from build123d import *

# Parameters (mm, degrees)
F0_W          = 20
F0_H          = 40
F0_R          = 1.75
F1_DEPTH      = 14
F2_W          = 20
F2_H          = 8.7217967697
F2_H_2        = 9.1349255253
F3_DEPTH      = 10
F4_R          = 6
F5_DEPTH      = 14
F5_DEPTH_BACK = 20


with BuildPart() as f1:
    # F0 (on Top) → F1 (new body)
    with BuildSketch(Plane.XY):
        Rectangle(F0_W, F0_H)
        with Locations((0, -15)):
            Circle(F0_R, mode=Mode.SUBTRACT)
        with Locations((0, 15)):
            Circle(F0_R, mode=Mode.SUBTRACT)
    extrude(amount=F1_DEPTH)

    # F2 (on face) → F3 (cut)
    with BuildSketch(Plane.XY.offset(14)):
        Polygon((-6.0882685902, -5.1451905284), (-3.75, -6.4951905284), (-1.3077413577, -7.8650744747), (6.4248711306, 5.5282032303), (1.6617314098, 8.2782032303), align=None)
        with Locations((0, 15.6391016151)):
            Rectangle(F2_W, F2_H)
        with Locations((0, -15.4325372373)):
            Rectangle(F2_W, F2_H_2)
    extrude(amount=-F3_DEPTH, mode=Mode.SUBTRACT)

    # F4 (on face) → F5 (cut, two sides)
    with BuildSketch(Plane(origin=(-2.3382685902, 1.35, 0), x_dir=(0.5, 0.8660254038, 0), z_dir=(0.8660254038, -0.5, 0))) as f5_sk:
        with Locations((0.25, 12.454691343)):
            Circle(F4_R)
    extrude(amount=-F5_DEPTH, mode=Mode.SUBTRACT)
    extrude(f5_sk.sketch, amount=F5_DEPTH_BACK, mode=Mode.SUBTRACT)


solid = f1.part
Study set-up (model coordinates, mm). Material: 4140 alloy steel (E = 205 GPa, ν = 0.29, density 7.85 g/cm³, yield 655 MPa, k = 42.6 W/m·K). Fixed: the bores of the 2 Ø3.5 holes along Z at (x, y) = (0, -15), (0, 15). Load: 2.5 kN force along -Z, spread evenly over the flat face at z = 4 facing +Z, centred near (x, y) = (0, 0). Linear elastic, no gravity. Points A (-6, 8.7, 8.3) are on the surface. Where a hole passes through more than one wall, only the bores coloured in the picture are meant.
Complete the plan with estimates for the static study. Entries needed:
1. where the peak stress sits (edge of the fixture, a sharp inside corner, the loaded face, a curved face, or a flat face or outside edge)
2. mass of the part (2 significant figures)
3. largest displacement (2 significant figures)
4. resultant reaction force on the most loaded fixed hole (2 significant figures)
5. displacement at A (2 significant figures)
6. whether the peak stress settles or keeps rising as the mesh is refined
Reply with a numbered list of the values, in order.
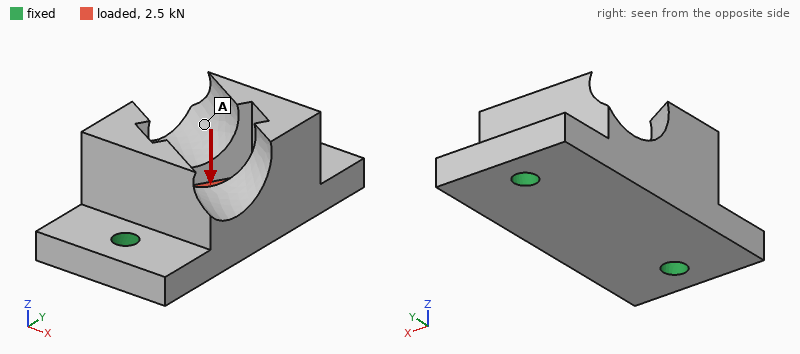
1. edge of the fixture
2. 42 g
3. 9.7 µm
4. 1.4 kN
5. 5.5 µm
6. keeps rising
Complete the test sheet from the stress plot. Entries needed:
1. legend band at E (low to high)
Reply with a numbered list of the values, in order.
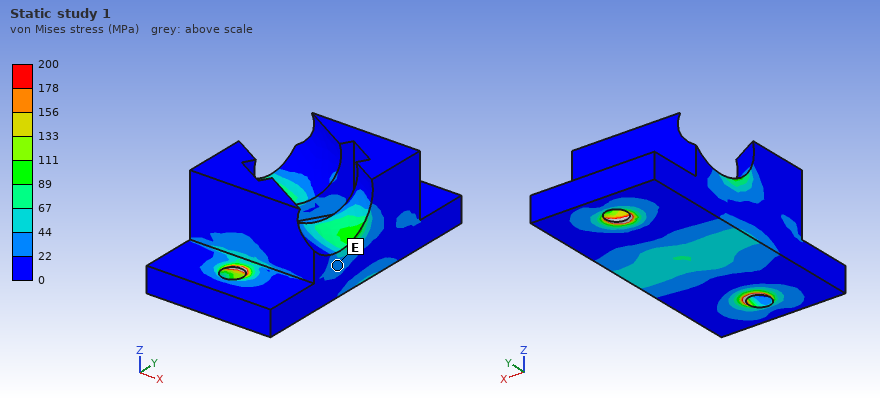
1. 22 to 44 MPa
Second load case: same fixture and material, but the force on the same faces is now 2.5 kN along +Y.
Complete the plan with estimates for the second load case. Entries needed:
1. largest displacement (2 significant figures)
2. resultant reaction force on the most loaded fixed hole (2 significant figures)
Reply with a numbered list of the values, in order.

1. 2.1 µm
2. 1.3 kN
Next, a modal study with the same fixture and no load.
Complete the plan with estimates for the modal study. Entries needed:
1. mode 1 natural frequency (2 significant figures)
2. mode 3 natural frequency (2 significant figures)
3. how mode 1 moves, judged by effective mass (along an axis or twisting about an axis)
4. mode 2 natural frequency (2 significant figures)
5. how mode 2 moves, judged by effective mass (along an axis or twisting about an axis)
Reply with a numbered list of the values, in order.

1. 12 kHz
2. 27 kHz
3. along X
4. 18 kHz
5. along Z
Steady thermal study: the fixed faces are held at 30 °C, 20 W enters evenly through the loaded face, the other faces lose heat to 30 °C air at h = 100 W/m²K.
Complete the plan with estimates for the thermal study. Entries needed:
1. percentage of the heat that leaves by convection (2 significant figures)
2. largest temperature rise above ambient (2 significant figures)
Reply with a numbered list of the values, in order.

1. 23 %
2. 40 K
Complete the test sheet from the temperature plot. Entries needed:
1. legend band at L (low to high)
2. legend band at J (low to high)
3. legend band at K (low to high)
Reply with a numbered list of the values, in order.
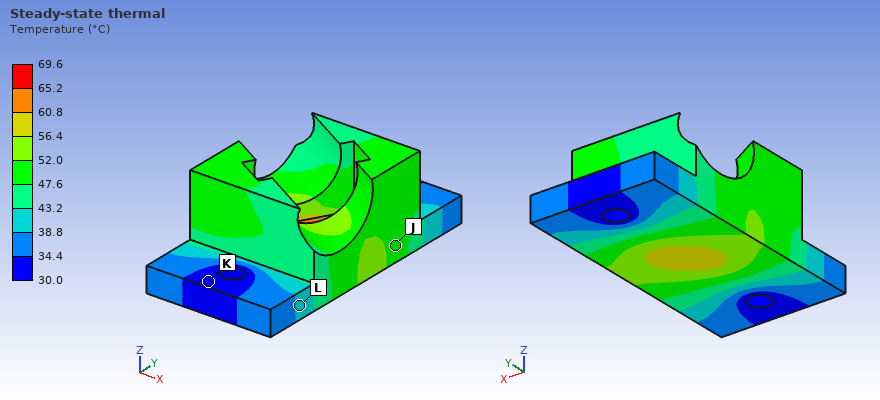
1. 38.8 to 43.2 °C
2. 47.6 to 52.0 °C
3. 30.0 to 34.4 °C
